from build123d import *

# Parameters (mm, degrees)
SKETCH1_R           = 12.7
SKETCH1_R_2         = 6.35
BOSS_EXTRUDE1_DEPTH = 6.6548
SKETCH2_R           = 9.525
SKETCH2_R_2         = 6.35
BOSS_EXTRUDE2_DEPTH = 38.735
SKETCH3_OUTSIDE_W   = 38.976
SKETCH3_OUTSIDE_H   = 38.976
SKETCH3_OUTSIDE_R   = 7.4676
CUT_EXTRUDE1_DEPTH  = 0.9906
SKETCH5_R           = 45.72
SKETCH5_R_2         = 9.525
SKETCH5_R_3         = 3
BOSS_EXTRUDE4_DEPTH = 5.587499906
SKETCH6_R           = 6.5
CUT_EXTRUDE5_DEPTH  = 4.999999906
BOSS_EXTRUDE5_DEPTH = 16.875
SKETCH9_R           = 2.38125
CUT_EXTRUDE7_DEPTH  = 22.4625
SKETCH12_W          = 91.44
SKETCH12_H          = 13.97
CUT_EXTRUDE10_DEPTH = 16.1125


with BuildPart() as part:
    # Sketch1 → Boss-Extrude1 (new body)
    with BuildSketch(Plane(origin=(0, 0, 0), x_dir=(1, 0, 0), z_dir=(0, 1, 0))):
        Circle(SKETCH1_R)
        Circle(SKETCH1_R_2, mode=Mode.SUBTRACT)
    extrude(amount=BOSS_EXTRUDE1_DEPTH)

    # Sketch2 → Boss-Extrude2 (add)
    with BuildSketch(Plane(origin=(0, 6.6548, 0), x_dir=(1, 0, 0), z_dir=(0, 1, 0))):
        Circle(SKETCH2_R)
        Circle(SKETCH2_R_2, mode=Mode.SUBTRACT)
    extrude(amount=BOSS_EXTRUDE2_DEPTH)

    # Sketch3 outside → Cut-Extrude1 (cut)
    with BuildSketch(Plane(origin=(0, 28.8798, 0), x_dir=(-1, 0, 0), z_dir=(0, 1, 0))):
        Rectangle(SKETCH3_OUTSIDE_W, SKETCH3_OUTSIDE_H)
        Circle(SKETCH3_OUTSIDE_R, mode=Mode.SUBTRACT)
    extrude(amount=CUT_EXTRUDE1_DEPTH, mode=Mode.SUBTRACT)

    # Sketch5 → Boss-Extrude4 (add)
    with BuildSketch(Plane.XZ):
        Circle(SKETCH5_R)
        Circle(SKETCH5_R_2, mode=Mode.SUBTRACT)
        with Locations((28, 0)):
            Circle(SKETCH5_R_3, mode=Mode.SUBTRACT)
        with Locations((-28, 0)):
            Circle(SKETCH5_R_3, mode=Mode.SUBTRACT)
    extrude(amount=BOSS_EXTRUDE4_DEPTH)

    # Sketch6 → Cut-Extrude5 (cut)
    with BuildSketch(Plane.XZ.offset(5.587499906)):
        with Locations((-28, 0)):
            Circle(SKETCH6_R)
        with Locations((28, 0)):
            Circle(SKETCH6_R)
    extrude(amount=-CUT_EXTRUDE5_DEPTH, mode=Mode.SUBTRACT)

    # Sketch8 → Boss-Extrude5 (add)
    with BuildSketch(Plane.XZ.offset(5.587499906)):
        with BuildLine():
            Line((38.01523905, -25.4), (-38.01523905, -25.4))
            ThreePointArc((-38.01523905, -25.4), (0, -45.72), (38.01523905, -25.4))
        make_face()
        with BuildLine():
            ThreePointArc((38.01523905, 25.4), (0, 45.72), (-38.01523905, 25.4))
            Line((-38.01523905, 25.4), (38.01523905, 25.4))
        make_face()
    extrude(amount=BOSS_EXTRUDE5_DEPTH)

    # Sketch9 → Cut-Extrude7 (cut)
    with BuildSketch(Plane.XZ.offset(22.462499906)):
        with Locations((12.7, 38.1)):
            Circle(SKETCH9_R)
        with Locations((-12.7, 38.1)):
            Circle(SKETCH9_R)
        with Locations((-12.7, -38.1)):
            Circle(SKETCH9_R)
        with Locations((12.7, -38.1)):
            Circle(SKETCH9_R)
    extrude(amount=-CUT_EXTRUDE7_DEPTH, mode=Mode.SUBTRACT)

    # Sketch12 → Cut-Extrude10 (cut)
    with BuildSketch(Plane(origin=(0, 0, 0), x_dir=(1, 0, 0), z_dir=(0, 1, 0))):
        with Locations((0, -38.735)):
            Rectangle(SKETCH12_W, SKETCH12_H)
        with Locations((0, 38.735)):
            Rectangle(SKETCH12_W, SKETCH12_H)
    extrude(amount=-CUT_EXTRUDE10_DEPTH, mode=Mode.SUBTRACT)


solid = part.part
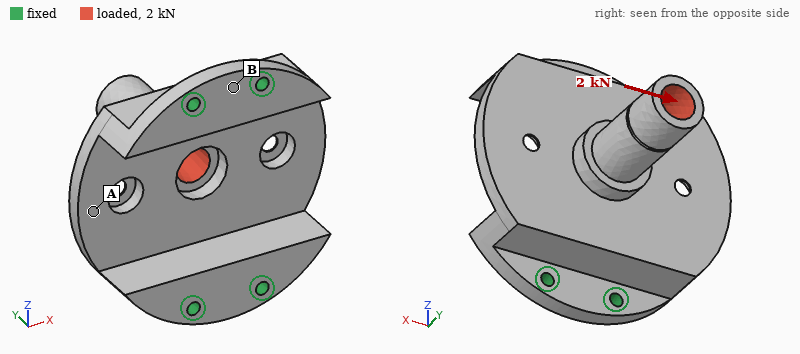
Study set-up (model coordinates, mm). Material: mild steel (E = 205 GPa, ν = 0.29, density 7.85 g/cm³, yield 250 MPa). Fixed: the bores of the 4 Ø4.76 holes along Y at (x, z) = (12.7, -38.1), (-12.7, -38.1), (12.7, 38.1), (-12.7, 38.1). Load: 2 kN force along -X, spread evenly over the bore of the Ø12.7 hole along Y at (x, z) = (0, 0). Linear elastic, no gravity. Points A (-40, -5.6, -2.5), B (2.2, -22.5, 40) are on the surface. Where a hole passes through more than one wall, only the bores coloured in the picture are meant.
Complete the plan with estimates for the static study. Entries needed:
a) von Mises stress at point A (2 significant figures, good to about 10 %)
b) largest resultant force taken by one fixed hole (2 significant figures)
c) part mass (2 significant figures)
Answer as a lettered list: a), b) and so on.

a) 21 MPa
b) 1.9 kN
c) 460 g
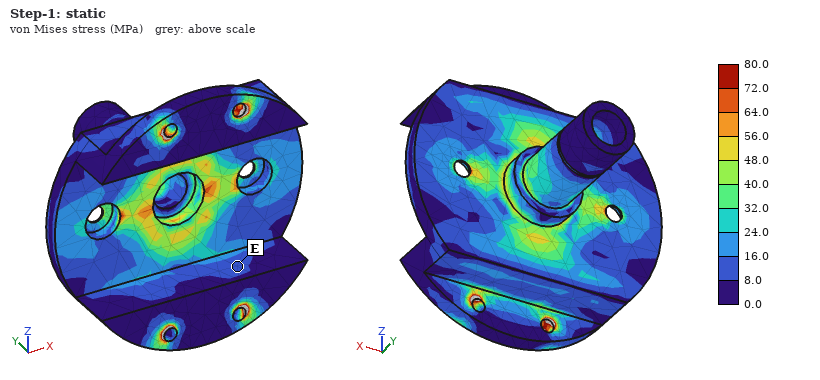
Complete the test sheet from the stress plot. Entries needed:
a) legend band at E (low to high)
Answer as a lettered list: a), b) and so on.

a) 8.0 to 16.0 MPa
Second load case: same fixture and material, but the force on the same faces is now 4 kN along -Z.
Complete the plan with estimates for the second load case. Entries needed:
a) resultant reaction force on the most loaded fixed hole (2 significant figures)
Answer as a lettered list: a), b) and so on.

a) 1.6 kN
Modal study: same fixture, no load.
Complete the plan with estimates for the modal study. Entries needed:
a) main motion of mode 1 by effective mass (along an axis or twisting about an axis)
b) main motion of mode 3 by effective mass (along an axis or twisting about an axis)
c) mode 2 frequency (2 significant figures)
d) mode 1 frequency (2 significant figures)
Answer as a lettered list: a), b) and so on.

a) along X
b) along Z
c) 4600 Hz
d) 3400 Hz
